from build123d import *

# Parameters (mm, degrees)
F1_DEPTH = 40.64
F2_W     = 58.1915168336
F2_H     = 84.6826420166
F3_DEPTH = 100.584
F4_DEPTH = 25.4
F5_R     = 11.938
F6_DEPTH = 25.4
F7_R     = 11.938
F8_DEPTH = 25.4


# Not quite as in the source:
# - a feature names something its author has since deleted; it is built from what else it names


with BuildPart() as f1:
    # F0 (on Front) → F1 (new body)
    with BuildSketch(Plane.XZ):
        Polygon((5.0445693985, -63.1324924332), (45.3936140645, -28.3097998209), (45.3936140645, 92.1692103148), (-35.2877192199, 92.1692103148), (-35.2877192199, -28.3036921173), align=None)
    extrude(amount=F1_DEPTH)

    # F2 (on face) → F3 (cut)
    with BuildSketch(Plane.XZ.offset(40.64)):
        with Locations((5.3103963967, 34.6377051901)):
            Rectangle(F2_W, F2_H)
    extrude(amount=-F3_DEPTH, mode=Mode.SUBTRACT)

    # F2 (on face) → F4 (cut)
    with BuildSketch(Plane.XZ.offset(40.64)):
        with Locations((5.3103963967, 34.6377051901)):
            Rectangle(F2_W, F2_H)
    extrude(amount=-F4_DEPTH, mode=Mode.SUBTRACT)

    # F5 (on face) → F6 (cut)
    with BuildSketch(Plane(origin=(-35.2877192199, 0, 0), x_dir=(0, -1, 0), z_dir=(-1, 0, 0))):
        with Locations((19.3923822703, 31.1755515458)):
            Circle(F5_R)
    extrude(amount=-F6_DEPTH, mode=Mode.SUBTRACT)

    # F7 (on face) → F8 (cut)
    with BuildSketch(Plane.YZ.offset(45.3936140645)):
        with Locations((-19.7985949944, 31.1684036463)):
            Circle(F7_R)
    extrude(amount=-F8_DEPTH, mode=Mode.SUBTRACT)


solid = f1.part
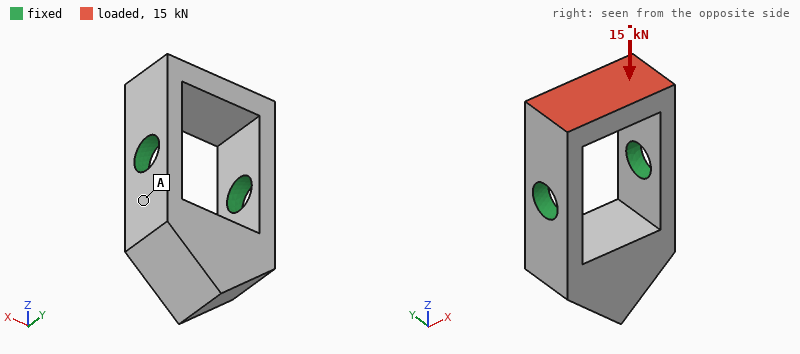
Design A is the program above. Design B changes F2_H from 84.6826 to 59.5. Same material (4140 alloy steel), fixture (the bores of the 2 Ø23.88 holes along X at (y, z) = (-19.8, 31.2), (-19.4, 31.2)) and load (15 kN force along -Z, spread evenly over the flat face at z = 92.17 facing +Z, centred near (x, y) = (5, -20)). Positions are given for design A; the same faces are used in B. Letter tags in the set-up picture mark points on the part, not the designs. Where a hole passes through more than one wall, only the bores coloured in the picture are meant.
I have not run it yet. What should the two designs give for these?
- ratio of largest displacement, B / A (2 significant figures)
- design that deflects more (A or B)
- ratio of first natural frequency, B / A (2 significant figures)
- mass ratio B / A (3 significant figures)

0.40
A
1.0
1.25
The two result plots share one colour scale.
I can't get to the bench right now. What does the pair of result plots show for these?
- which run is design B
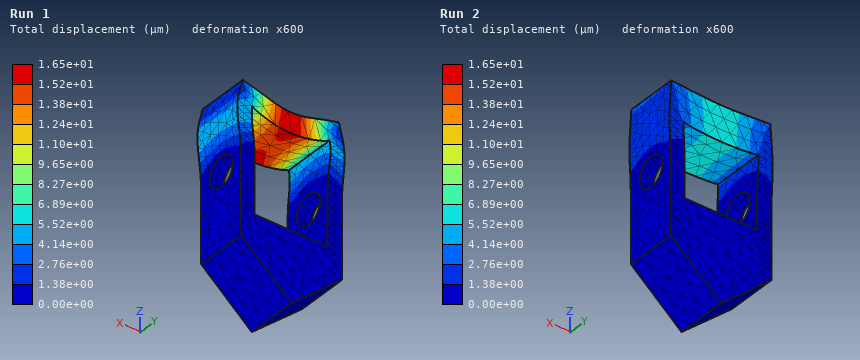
Run 2
